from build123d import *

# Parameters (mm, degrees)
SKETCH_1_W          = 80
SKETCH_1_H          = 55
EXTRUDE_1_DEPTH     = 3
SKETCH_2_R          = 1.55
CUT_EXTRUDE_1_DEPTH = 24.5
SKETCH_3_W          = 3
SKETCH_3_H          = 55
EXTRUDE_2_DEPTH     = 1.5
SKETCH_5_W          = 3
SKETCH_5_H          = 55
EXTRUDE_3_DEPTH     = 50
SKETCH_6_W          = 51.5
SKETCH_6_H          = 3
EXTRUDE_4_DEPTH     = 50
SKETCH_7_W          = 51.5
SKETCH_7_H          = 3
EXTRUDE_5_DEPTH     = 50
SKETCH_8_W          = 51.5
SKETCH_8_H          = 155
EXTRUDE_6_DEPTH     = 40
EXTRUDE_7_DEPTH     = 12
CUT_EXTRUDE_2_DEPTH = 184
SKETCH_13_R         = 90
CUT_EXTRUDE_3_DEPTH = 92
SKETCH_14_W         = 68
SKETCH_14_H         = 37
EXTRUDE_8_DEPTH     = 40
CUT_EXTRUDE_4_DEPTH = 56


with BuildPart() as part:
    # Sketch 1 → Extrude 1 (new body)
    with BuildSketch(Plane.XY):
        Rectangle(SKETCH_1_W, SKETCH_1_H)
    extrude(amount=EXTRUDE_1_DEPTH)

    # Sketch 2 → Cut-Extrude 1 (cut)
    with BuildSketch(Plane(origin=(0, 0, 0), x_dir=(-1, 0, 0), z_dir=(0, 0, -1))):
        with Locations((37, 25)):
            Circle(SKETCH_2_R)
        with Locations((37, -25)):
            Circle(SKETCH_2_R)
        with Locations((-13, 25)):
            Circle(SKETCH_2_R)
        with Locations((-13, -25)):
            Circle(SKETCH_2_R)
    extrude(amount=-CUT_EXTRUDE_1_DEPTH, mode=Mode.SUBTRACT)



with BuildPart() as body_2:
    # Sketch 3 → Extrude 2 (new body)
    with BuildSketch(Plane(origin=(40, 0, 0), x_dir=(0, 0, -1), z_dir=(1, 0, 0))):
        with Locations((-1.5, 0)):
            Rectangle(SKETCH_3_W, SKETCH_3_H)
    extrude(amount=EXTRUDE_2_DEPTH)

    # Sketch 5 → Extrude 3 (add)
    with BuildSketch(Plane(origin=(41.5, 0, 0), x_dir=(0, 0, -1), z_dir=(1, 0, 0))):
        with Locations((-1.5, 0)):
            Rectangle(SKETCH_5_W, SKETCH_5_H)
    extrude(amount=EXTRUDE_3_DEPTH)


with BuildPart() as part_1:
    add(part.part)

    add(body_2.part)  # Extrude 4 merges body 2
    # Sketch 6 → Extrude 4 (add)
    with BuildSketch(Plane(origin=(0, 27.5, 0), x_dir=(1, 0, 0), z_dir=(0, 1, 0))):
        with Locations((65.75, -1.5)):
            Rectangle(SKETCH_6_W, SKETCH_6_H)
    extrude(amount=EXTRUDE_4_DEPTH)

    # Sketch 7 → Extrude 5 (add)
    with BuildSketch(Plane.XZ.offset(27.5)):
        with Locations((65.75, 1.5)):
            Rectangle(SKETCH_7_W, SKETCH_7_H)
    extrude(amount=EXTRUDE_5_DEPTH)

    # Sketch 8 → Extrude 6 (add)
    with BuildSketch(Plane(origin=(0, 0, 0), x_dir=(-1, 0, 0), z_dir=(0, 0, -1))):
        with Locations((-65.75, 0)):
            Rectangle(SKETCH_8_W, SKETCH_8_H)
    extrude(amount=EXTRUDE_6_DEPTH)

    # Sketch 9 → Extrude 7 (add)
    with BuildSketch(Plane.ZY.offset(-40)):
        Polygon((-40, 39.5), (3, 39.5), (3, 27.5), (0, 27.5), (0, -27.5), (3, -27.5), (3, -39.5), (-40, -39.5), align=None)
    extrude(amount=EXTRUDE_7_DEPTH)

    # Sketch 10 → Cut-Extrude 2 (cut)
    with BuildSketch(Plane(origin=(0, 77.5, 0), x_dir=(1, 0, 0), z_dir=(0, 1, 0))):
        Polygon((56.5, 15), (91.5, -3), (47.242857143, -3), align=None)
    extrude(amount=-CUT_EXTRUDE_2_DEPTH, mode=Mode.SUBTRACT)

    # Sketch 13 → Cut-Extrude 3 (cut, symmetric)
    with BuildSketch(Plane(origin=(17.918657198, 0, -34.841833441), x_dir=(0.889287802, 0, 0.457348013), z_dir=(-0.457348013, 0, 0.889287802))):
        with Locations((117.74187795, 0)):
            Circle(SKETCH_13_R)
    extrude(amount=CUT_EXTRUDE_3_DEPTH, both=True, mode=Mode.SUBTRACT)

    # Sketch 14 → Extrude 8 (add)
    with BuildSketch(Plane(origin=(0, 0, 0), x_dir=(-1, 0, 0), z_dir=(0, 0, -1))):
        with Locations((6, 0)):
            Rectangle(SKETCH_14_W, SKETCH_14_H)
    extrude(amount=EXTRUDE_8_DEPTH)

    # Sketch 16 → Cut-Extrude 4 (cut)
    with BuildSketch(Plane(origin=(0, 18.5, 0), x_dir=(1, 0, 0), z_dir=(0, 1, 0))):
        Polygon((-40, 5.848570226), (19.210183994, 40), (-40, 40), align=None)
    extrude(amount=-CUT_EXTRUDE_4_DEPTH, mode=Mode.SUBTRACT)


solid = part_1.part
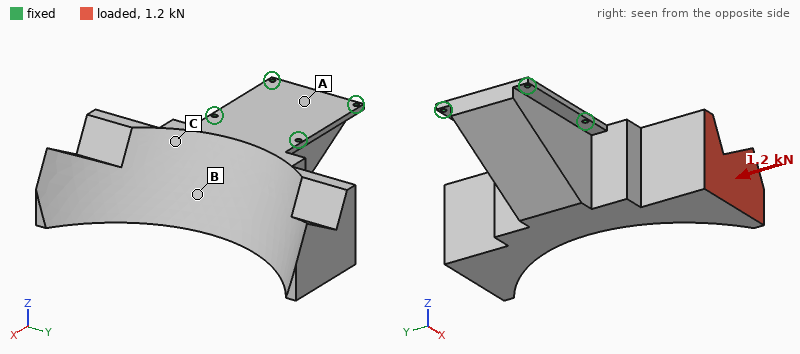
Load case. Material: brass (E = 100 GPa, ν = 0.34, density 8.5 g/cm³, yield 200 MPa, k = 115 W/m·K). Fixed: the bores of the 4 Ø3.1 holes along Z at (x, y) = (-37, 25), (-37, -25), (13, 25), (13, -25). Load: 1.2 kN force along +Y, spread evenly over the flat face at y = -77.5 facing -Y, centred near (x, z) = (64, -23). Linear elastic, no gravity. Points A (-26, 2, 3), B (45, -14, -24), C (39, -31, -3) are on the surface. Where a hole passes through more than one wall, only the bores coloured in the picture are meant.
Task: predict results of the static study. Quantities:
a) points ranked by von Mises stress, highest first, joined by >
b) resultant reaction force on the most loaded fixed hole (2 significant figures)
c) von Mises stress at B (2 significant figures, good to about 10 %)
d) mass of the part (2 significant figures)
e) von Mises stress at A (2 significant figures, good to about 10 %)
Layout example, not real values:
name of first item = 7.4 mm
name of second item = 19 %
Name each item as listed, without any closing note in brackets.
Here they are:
points ranked by von Mises stress, highest first, joined by > = B > C > A
resultant reaction force on the most loaded fixed hole = 1.2 kN
von Mises stress at B = 16 MPa
mass of the part = 1.8 kg
von Mises stress at A = 4.2 MPa
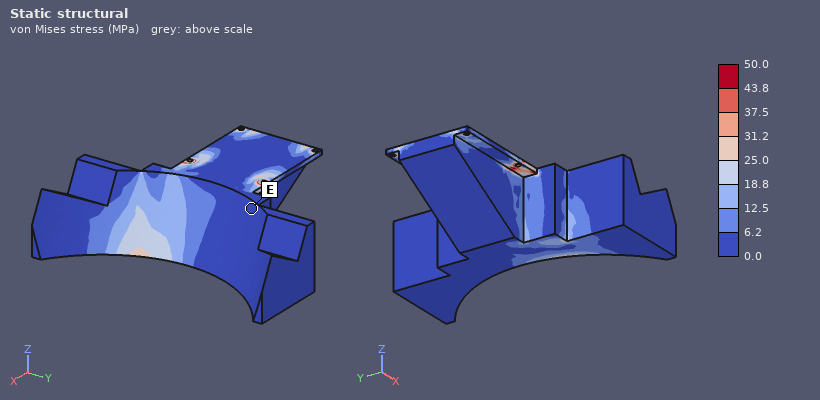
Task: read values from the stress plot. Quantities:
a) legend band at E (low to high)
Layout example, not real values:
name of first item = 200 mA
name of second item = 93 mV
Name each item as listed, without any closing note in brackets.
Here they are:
legend band at E = 0.0 to 6.2 MPa
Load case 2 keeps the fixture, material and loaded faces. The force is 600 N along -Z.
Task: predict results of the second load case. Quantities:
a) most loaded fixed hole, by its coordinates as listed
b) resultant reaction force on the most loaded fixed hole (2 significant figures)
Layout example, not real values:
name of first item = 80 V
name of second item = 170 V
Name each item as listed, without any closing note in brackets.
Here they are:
most loaded fixed hole, by its coordinates as listed = (13, -25)
resultant reaction force on the most loaded fixed hole = 1.3 kN
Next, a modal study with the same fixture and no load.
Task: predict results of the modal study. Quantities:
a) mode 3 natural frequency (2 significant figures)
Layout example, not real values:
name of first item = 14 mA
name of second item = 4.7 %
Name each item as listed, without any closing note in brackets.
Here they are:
mode 3 natural frequency = 920 Hz
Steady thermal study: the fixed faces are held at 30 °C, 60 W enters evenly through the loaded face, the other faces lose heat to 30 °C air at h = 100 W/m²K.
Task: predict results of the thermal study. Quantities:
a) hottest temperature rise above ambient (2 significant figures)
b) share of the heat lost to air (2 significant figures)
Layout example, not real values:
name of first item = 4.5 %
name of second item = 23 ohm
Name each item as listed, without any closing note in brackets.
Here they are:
hottest temperature rise above ambient = 55 K
share of the heat lost to air = 76 %
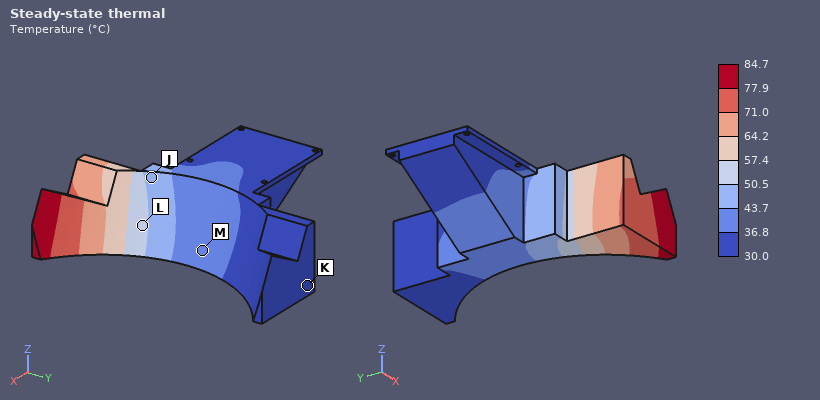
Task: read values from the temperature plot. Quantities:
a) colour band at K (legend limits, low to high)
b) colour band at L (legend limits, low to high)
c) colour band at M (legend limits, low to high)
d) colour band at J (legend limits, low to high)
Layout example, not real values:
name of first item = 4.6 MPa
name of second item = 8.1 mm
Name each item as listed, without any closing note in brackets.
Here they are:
colour band at K = 30.0 to 36.8 °C
colour band at L = 50.5 to 57.4 °C
colour band at M = 36.8 to 43.7 °C
colour band at J = 43.7 to 50.5 °C
